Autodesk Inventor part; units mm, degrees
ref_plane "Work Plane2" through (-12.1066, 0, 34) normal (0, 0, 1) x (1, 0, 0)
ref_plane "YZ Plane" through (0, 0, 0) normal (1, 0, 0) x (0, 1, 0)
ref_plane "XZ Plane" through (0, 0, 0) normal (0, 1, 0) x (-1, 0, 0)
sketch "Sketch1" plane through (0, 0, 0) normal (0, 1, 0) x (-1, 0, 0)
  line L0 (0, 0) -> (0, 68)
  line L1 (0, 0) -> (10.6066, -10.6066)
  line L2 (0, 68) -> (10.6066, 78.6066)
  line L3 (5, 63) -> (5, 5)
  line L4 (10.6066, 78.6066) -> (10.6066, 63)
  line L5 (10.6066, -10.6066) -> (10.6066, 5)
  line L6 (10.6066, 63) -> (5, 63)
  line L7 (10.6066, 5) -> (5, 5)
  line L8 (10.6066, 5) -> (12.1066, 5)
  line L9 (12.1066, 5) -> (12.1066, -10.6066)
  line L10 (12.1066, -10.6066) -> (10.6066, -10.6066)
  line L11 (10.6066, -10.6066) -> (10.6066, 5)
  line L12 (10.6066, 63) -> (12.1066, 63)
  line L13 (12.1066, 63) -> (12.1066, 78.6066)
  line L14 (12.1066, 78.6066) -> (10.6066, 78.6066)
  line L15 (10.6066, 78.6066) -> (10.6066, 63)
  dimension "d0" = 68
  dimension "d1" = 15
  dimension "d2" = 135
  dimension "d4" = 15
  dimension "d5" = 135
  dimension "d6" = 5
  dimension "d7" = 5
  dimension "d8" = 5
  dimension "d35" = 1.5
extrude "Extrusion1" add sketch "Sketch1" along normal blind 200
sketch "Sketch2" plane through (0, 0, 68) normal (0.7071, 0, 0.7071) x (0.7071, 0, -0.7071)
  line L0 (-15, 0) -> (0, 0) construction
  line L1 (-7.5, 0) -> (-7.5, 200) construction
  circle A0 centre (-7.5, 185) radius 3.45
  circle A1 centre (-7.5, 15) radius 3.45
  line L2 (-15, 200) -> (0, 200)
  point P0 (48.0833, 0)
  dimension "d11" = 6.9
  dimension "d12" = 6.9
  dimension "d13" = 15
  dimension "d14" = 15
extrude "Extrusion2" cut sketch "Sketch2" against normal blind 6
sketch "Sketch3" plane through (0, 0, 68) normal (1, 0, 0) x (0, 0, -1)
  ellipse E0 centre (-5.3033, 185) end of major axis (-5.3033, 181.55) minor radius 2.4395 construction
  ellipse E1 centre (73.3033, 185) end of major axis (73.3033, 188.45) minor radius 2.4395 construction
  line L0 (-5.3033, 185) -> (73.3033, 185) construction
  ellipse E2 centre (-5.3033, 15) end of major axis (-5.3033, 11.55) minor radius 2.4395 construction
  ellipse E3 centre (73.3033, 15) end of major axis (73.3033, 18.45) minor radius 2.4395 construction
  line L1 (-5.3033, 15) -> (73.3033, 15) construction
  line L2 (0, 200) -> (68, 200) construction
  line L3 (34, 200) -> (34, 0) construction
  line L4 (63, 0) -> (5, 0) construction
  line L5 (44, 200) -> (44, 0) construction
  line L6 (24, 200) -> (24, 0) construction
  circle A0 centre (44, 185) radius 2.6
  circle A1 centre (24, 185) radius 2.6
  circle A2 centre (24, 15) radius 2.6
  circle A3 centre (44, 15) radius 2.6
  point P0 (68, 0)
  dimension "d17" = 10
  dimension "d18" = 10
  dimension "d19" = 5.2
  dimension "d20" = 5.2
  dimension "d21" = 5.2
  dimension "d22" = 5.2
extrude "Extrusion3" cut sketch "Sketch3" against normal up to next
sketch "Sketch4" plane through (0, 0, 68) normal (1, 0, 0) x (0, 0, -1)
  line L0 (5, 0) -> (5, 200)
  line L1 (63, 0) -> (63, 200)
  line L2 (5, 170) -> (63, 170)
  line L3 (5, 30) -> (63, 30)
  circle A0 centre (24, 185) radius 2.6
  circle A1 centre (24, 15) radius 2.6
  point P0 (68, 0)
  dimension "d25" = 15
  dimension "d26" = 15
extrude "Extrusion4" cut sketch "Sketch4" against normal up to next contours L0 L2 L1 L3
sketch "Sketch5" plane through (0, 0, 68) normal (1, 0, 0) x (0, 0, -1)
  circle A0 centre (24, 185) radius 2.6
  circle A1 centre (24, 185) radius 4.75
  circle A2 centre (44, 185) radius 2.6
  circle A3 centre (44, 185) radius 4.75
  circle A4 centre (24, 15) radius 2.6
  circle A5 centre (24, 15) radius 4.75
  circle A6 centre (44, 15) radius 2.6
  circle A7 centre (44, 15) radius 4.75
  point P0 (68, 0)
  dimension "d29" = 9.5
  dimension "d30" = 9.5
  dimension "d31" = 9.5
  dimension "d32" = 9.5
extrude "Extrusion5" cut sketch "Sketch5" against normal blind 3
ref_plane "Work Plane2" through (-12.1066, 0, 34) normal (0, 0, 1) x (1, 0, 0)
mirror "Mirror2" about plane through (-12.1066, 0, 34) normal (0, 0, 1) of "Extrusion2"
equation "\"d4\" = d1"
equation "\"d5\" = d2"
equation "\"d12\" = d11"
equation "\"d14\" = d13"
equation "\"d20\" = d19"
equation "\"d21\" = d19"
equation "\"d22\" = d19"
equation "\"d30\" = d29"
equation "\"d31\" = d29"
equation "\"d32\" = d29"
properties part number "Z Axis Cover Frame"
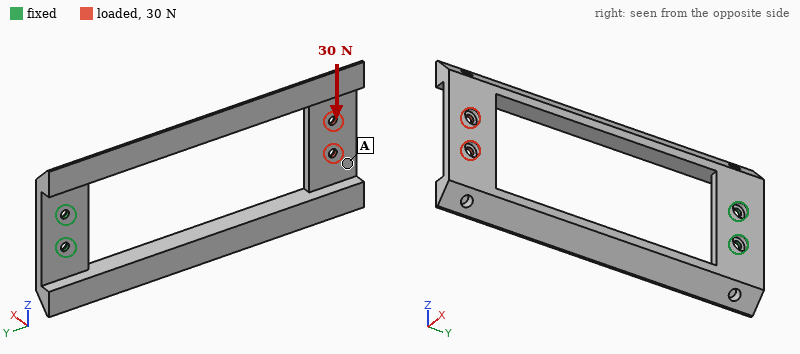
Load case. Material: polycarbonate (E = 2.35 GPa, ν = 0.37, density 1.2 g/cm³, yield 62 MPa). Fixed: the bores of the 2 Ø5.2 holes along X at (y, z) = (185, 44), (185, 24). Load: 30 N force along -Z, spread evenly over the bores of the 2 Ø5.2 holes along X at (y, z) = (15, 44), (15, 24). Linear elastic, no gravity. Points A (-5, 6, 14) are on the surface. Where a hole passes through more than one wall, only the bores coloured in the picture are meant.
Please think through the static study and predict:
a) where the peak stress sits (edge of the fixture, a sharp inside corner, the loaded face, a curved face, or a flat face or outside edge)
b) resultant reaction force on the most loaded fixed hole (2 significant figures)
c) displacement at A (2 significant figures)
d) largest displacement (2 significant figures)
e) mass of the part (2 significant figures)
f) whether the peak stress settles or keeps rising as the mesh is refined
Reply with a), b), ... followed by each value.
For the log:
a) edge of the fixture
b) 220 N
c) 2.1 mm
d) 2.2 mm
e) 82 g
f) keeps rising
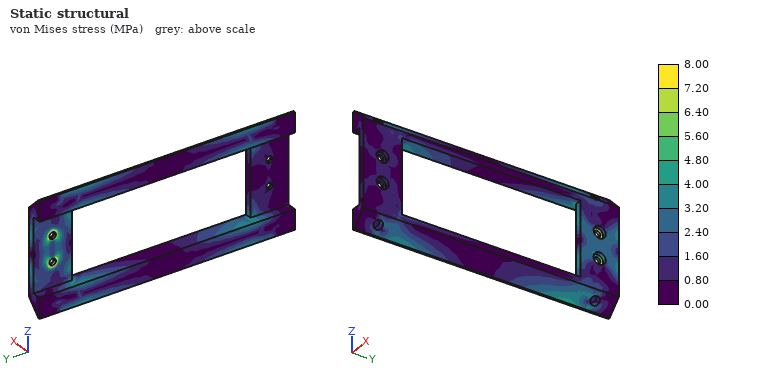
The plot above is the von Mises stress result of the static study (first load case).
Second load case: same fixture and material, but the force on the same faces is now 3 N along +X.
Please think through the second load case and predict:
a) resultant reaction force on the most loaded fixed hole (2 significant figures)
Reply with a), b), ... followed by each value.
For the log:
a) 2.1 N
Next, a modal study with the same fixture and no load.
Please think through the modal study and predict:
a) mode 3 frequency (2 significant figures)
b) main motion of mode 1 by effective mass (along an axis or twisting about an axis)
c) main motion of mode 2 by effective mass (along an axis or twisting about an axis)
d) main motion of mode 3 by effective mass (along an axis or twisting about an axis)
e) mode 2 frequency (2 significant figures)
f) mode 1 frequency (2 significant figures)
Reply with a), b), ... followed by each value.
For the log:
a) 120 Hz
b) along X
c) along Z
d) along Z
e) 100 Hz
f) 34 Hz
